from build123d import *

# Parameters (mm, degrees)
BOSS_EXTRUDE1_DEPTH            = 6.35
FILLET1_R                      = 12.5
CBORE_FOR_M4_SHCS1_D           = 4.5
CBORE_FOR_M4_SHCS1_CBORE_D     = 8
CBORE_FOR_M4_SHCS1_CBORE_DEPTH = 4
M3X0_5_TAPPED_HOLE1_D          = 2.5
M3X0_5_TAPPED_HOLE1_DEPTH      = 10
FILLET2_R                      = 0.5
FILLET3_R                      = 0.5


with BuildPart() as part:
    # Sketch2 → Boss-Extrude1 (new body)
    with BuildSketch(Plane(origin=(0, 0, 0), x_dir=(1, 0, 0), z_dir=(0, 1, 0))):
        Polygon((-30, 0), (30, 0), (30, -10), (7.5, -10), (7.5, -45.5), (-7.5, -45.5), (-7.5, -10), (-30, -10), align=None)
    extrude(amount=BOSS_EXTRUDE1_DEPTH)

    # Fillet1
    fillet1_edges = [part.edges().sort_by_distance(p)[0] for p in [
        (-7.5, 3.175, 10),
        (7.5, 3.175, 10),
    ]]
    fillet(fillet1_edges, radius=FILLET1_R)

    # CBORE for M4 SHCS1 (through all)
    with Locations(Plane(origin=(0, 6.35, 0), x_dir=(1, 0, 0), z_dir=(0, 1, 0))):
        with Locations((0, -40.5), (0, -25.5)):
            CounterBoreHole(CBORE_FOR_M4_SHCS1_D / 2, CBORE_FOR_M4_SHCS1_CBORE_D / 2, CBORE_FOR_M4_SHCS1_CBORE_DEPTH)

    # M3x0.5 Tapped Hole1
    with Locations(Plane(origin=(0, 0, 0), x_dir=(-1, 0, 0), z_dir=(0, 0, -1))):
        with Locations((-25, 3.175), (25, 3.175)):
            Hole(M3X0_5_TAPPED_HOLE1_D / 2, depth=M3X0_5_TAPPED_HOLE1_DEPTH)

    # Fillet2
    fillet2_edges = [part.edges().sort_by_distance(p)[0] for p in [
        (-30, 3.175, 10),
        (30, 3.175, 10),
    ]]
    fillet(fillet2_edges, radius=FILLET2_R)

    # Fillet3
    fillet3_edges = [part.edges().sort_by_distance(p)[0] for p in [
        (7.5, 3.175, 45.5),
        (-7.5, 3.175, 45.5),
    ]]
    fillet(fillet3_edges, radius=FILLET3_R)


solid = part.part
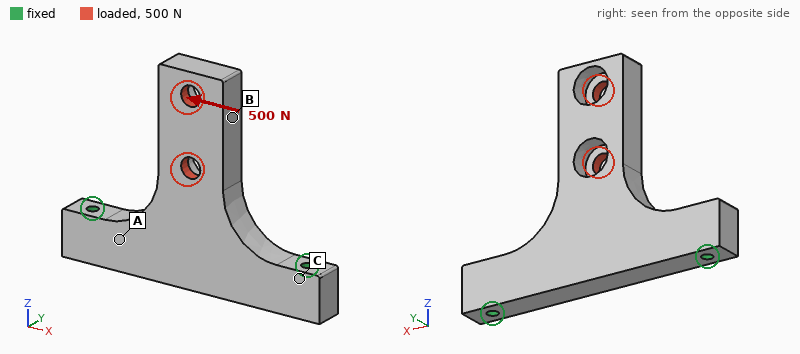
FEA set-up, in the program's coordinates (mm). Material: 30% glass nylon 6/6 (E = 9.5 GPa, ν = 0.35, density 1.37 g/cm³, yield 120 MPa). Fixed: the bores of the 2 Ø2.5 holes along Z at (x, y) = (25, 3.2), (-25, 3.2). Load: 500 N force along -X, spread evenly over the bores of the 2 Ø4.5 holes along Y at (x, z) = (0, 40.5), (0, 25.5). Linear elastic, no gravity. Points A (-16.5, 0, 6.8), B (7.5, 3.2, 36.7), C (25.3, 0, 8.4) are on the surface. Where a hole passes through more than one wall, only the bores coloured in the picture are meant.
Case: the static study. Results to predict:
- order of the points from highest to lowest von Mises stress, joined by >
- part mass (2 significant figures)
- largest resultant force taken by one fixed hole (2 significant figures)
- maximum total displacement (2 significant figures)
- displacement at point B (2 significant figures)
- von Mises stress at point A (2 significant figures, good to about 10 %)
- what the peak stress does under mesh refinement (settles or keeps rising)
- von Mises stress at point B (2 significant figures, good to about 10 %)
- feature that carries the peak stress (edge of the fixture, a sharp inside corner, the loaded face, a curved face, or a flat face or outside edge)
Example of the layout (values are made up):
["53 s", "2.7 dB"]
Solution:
["A > B > C", "9.6 g", "430 N", "0.32 mm", "0.22 mm", "12 MPa", "keeps rising", "7.6 MPa", "edge of the fixture"]
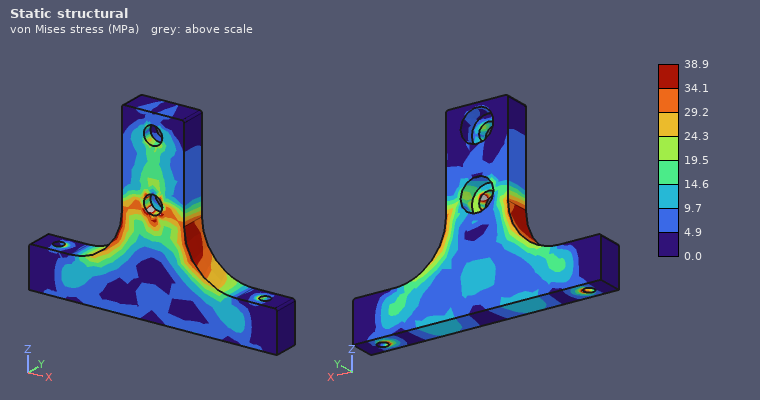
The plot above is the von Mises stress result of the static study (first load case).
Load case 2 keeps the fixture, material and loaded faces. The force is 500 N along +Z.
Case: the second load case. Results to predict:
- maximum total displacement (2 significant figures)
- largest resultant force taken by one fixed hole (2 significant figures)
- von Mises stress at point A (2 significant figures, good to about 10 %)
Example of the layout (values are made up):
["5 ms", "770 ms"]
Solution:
["0.35 mm", "280 N", "18 MPa"]
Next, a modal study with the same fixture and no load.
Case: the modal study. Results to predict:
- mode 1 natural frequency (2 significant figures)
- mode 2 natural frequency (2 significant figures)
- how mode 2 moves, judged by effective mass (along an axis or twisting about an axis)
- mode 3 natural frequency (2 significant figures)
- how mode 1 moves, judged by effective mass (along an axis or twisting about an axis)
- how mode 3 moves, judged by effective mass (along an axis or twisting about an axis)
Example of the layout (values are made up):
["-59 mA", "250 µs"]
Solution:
["1300 Hz", "4700 Hz", "along X", "4900 Hz", "along Y", "along Y"]
